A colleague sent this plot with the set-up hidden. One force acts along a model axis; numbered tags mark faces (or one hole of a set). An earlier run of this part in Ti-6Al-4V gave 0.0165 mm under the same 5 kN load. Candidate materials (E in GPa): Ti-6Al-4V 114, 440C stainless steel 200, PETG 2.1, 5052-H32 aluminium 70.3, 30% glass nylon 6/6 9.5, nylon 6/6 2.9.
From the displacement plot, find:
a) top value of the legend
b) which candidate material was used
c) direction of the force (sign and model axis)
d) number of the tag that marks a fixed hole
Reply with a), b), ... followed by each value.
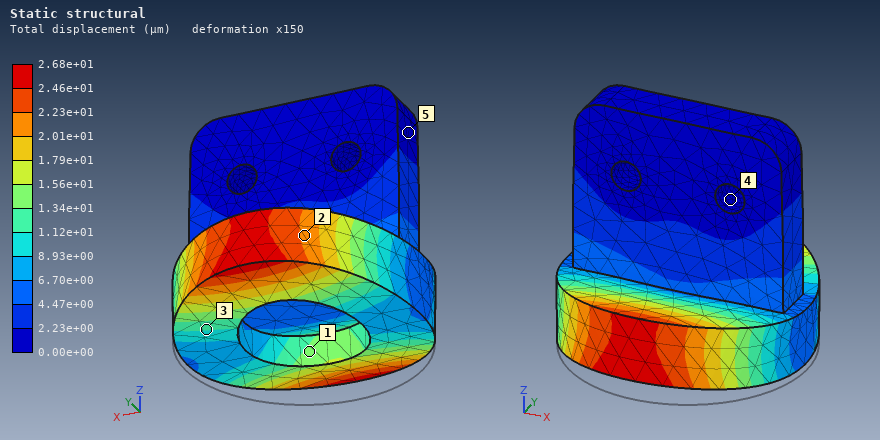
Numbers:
a) 2.68e+01 µm
b) 5052-H32 aluminium
c) +Z
d) 4
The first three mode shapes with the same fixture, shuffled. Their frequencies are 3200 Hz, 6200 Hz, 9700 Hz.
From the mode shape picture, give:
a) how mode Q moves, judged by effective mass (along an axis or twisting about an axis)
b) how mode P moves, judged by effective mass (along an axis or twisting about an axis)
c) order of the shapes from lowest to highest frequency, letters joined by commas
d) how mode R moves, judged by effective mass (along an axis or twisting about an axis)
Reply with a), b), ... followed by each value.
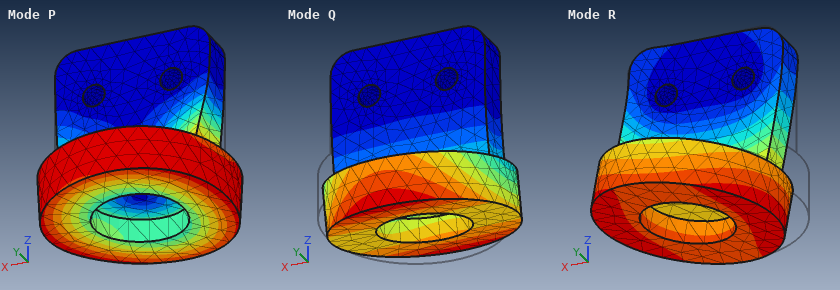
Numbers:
a) along Y
b) twisting about Z
c) Q, P, R
d) along X
